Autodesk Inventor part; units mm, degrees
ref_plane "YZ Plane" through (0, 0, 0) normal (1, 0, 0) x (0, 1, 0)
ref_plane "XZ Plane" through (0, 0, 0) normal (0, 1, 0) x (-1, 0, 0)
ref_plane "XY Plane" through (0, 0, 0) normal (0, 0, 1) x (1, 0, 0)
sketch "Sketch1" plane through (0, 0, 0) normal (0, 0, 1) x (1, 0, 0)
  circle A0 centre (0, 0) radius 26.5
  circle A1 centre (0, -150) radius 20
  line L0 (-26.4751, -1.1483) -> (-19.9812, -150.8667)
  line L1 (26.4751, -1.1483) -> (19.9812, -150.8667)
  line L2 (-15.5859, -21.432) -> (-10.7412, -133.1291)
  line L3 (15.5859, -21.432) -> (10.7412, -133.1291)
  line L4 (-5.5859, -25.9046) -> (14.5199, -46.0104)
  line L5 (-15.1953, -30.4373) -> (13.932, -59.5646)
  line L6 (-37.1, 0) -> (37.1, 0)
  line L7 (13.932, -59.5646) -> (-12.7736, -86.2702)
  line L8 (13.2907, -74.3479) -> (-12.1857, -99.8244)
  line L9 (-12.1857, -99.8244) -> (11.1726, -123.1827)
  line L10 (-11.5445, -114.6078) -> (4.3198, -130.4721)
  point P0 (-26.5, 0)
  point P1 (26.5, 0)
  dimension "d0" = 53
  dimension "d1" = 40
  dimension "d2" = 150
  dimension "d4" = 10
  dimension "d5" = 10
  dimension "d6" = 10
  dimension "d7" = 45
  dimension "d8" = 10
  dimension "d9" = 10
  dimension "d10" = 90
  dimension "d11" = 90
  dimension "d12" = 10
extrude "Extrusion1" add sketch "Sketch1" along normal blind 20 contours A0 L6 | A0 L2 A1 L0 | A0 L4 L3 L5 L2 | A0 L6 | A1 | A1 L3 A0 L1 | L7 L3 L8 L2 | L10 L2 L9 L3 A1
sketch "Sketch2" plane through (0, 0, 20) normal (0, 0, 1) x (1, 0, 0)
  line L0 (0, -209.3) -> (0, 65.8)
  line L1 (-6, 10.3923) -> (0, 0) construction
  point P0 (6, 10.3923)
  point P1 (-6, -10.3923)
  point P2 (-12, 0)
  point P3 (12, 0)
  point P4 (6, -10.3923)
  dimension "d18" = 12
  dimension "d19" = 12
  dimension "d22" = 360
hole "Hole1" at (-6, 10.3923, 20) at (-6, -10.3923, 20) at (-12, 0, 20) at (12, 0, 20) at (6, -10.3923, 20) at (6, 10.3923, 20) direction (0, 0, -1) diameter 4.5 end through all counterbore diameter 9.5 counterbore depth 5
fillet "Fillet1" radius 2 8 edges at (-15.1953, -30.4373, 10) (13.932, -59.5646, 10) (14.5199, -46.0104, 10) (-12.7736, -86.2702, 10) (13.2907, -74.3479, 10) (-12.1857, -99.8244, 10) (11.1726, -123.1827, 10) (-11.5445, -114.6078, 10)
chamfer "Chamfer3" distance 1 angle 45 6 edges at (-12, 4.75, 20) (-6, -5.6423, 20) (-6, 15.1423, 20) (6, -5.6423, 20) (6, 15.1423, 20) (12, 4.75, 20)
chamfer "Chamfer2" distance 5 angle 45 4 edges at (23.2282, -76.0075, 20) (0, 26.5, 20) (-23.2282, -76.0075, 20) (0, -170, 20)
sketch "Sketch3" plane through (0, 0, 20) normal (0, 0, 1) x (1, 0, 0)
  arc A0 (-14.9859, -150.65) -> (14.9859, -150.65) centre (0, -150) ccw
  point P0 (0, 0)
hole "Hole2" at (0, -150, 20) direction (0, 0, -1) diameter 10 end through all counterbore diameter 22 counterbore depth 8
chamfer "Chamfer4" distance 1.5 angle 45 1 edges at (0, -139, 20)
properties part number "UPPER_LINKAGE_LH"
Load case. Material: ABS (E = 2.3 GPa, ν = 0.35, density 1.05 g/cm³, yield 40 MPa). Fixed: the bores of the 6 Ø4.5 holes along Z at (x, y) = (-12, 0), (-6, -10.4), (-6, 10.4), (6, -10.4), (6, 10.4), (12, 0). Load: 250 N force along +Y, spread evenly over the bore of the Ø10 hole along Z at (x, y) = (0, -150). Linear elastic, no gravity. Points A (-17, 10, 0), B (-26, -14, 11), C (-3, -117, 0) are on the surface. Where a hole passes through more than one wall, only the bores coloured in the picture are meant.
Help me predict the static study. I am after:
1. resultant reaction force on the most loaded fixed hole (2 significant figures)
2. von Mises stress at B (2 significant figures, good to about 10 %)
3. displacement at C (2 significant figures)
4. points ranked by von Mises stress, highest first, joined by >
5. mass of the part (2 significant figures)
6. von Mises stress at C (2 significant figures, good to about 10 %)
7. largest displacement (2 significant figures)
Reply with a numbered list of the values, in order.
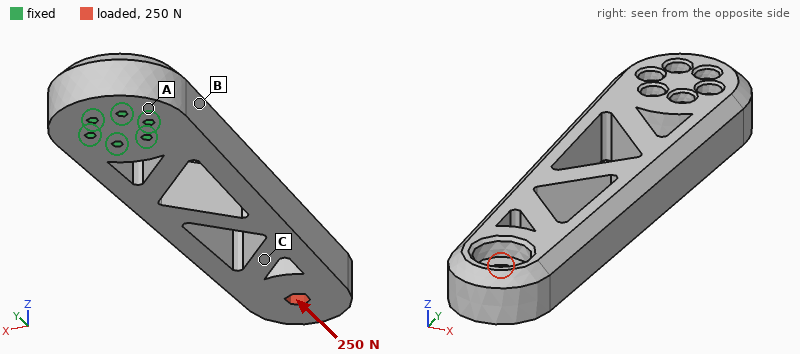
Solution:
1. 63 N
2. 0.34 MPa
3. 0.16 mm
4. C > B > A
5. 130 g
6. 0.62 MPa
7. 0.33 mm
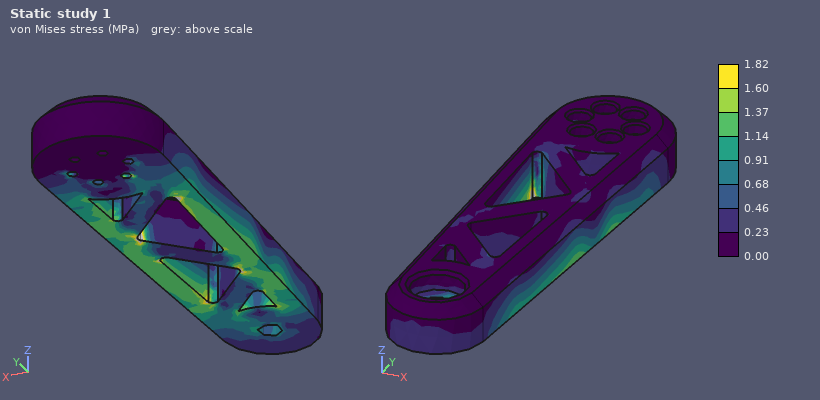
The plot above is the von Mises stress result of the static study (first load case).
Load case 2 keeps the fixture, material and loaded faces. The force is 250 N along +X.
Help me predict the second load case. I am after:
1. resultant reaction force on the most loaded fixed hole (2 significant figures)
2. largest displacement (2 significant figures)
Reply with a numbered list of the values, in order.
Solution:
1. 630 N
2. 1.2 mm
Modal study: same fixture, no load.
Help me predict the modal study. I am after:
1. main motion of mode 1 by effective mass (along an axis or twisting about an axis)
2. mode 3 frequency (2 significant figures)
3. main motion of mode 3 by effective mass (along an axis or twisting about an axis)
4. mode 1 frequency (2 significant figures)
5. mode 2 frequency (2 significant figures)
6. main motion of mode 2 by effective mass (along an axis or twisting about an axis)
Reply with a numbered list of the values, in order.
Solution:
1. along Z
2. 800 Hz
3. twisting about Y
4. 160 Hz
5. 410 Hz
6. along X
